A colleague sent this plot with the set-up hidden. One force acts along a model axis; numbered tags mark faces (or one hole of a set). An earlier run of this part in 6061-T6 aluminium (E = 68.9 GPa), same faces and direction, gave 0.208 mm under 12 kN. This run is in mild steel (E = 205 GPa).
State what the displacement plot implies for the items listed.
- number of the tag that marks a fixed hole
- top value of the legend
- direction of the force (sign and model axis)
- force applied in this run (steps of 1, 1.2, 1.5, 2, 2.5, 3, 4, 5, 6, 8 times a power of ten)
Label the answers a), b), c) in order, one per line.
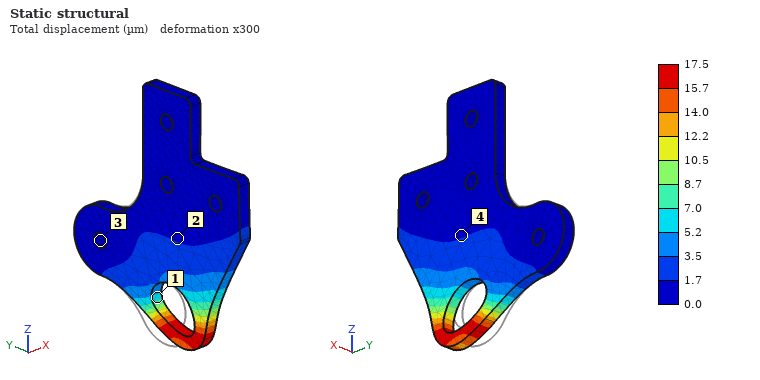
a) 3
b) 17.5 µm
c) -Y
d) 3 kN
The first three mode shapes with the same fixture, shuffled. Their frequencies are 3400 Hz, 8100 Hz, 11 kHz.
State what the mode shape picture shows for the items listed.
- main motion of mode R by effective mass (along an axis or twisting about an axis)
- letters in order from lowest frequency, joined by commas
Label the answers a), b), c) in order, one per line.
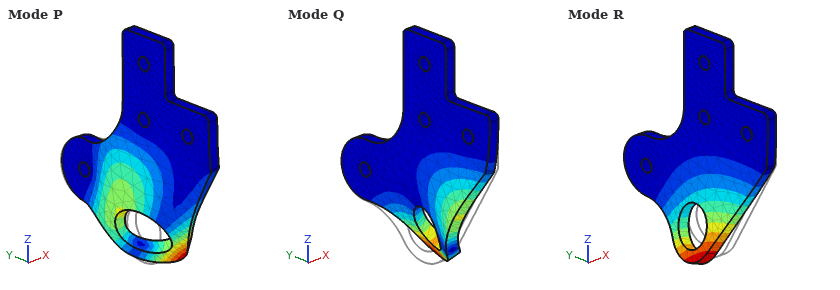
a) along X
b) R, Q, P
